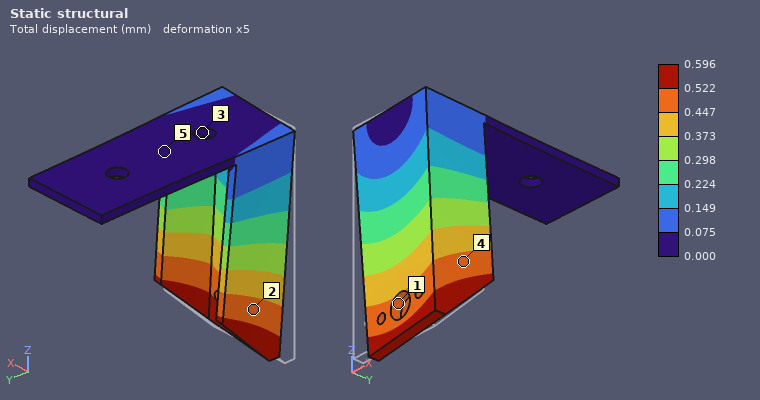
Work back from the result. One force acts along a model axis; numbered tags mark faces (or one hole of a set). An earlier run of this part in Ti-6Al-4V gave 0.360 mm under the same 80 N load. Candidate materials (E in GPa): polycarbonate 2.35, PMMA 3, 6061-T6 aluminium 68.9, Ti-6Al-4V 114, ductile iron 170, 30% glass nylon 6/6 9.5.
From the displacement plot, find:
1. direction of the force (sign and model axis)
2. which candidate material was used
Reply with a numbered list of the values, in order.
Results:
1. +X
2. 6061-T6 aluminium
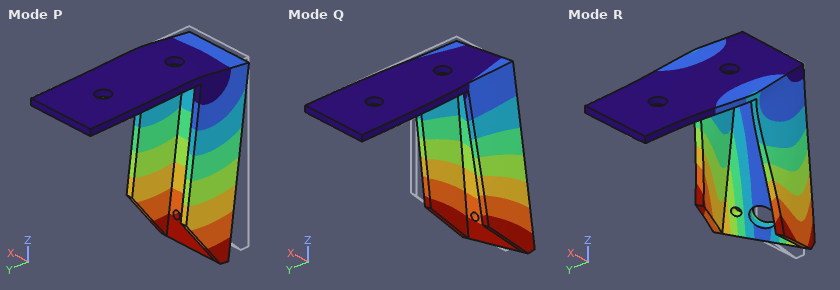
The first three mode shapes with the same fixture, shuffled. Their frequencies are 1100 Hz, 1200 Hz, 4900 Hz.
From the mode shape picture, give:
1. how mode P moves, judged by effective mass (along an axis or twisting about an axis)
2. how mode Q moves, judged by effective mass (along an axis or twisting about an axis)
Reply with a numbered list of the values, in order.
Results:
1. along Y
2. along X
